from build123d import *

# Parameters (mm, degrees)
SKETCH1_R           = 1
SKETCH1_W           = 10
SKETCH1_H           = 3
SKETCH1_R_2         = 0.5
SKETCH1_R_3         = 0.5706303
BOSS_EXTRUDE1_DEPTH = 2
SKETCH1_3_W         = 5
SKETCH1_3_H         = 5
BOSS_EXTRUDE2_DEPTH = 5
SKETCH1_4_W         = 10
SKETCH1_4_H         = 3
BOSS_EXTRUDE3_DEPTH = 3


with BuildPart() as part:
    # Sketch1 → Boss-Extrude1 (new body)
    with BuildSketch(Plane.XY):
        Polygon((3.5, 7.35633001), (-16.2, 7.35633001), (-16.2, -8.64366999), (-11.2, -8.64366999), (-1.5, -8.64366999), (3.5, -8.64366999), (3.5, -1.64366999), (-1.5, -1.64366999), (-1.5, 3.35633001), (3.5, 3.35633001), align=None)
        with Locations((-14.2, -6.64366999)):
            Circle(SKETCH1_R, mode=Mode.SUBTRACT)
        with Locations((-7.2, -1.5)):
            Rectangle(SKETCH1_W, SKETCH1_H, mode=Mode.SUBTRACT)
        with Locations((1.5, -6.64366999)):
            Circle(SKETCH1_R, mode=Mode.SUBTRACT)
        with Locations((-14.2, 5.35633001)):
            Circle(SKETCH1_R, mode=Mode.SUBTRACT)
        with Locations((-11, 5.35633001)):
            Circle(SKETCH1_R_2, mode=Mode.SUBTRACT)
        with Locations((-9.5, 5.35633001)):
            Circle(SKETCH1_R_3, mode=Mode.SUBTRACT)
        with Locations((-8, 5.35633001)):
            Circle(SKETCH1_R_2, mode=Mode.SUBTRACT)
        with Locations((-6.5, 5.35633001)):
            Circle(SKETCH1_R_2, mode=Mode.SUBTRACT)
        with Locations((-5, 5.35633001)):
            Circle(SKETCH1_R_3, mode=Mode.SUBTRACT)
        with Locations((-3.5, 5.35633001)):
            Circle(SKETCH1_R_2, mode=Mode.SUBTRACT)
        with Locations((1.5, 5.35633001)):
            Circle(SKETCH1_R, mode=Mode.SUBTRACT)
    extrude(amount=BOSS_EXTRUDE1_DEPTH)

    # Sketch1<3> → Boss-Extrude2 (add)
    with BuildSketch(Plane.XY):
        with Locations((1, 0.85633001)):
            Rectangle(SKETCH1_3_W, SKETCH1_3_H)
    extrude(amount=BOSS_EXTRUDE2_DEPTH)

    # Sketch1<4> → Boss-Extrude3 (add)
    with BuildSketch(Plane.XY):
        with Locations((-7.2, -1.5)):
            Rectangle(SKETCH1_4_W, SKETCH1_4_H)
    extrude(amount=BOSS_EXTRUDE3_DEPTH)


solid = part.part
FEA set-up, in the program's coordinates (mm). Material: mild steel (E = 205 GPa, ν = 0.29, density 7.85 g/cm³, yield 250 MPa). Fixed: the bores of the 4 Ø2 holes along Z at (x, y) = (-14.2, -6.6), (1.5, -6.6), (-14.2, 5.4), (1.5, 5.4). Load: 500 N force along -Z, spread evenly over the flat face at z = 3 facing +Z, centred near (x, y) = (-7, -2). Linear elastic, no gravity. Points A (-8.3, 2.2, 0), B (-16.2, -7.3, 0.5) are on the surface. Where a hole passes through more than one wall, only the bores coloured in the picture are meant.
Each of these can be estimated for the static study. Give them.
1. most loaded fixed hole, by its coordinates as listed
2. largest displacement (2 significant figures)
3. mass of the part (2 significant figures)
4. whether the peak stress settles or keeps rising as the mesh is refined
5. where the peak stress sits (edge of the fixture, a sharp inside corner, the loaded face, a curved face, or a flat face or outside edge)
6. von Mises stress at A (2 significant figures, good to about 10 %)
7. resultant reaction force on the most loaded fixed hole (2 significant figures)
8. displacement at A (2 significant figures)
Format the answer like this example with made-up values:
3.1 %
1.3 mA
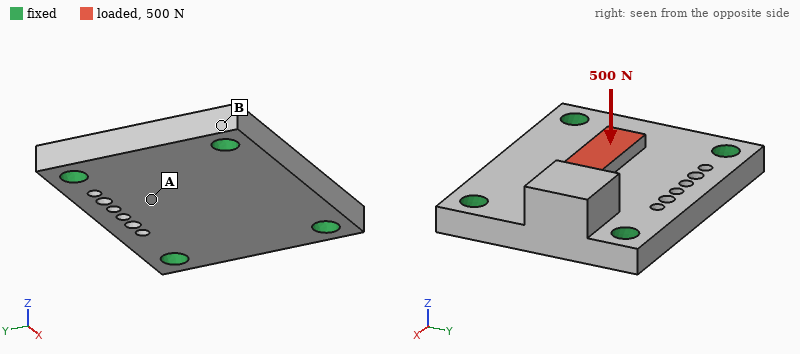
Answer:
(-14.2, -6.6)
5.4 µm
5.5 g
keeps rising
edge of the fixture
36 MPa
160 N
4.1 µm
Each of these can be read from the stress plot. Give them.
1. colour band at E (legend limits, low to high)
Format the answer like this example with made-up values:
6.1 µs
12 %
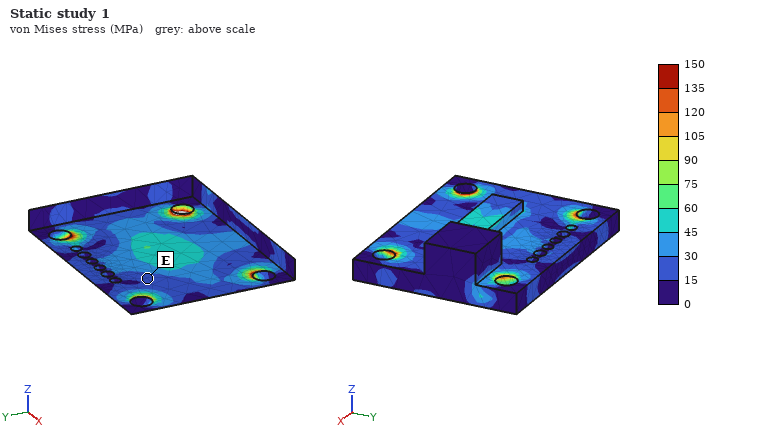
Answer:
15 to 30 MPa
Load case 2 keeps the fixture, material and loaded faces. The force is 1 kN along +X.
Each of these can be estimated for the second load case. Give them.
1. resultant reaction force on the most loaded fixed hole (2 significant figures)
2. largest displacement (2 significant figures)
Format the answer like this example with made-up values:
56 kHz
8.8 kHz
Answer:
330 N
3.2 µm
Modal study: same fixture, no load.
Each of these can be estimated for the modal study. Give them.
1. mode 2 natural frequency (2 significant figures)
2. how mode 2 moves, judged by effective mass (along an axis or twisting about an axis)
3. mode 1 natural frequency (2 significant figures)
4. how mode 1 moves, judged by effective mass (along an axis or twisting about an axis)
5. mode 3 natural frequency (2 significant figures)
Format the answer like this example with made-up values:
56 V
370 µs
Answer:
51 kHz
twisting about X
35 kHz
along Z
58 kHz
